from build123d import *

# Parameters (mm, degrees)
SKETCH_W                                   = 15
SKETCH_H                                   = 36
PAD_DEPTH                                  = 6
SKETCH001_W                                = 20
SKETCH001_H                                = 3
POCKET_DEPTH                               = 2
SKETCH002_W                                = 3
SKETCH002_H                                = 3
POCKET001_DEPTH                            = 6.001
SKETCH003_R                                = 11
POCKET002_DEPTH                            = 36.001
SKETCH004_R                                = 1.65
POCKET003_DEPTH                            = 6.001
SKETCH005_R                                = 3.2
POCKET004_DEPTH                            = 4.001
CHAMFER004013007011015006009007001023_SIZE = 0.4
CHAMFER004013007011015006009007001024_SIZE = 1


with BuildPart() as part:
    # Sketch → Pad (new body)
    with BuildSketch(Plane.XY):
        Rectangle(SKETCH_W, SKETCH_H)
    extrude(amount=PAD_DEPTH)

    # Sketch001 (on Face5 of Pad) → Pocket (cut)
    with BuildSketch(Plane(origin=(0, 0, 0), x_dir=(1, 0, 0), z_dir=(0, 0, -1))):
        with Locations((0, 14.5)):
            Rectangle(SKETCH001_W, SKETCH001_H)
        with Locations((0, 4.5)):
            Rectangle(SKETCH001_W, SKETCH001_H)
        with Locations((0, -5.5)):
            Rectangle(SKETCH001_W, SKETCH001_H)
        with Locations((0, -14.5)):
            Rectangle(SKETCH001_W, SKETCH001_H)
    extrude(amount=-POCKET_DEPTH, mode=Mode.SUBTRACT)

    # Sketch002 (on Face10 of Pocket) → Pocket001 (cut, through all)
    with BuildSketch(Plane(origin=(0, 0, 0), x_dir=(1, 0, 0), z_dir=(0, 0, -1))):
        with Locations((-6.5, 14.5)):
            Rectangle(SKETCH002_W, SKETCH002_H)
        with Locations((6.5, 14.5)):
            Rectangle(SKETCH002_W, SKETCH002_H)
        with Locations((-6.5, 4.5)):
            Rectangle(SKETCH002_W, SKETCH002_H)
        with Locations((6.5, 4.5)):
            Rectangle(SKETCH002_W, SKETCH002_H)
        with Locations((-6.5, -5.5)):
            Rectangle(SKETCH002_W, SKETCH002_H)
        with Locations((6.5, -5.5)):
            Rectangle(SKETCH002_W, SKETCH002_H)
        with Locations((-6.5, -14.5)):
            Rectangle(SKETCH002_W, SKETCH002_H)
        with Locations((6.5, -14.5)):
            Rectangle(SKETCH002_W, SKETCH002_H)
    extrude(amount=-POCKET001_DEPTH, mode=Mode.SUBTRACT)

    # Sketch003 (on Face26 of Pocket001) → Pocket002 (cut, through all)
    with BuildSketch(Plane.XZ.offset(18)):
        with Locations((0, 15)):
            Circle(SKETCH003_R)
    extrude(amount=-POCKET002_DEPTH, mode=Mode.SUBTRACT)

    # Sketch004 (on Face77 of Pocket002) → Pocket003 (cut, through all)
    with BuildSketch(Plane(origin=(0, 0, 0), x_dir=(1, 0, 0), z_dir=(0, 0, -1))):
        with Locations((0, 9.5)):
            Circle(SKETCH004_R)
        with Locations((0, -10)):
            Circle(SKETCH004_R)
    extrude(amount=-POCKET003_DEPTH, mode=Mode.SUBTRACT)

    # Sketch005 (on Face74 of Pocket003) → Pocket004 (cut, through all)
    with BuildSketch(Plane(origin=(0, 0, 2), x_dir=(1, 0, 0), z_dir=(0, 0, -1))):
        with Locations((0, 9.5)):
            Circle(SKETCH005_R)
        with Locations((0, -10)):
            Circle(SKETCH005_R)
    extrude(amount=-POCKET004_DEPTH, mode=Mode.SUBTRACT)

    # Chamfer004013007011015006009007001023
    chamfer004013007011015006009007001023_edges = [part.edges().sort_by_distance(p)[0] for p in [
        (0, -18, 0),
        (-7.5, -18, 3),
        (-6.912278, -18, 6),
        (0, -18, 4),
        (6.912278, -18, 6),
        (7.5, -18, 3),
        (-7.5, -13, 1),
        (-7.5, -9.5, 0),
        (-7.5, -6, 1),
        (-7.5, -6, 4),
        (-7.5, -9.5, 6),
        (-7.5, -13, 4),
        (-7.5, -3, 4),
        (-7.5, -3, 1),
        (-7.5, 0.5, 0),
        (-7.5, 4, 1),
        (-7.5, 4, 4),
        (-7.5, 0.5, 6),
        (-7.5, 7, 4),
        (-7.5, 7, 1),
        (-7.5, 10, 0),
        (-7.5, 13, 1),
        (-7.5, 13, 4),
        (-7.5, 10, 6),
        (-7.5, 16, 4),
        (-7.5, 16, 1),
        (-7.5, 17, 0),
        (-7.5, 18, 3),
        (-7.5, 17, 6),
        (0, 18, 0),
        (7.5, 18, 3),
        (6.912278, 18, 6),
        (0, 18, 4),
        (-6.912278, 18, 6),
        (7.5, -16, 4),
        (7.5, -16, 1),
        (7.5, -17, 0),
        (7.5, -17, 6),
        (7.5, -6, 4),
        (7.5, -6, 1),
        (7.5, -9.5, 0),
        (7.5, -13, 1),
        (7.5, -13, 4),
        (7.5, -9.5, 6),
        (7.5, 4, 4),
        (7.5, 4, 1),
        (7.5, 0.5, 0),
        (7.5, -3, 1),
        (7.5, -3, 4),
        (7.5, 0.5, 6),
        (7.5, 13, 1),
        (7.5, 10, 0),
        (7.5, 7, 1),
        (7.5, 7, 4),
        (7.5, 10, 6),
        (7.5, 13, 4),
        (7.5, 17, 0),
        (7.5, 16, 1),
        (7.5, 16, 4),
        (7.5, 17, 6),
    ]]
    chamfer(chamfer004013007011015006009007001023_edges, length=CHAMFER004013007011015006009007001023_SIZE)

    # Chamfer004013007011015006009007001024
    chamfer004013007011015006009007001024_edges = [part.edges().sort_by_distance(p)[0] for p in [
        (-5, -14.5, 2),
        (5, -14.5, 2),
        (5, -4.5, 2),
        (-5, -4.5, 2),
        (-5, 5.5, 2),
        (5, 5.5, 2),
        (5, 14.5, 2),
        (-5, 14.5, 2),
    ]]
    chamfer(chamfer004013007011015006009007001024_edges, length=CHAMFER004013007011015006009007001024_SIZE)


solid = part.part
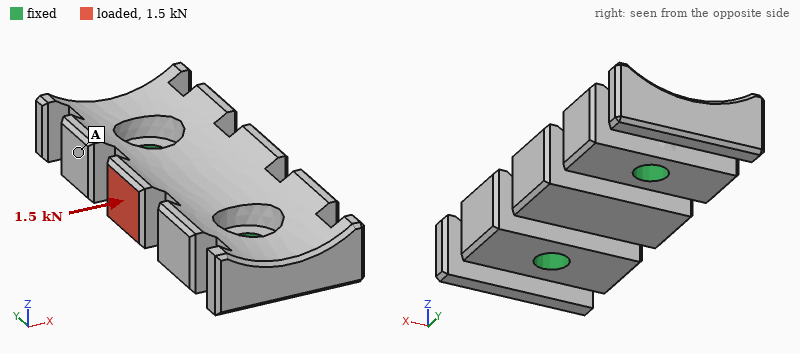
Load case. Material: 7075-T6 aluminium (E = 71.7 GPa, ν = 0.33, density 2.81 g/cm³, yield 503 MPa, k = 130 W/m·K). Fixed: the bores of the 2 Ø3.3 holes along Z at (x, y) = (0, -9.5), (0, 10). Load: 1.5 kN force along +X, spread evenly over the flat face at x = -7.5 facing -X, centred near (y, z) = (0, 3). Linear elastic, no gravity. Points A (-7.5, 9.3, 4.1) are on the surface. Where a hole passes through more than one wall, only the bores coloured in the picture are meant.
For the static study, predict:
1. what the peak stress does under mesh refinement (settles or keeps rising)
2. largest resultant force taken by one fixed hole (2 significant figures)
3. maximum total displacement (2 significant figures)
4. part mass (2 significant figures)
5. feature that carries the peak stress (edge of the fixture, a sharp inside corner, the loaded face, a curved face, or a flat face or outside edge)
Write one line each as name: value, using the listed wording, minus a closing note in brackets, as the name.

what the peak stress does under mesh refinement: keeps rising
largest resultant force taken by one fixed hole: 760 N
maximum total displacement: 41 µm
part mass: 5.1 g
feature that carries the peak stress: a sharp inside corner
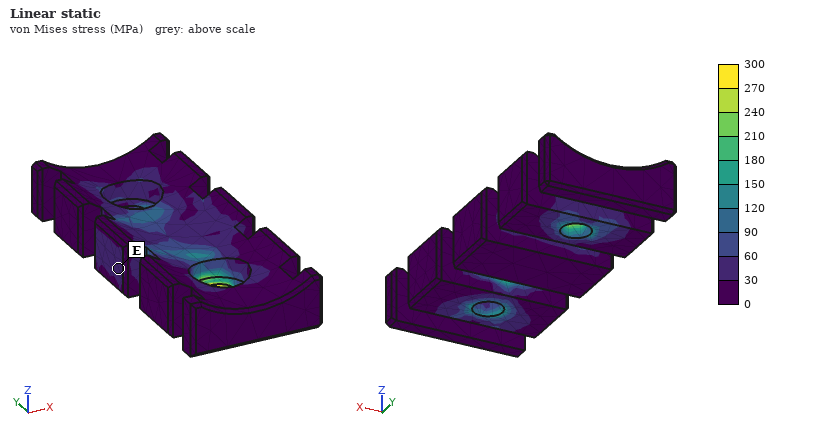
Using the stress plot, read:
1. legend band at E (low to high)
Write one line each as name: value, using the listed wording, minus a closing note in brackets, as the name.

legend band at E: 30 to 60 MPa
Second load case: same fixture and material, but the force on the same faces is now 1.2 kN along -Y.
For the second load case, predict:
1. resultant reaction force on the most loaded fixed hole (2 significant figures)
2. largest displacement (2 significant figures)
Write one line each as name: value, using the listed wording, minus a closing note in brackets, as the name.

resultant reaction force on the most loaded fixed hole: 770 N
largest displacement: 32 µm
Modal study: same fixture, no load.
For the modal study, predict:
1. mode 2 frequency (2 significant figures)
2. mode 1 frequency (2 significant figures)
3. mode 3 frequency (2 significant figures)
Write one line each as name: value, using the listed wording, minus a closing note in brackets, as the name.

mode 2 frequency: 20 kHz
mode 1 frequency: 17 kHz
mode 3 frequency: 21 kHz
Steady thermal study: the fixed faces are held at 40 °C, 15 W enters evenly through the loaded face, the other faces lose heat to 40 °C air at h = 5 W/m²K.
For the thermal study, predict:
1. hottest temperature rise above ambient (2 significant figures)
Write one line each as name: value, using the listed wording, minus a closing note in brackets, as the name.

hottest temperature rise above ambient: 38 K
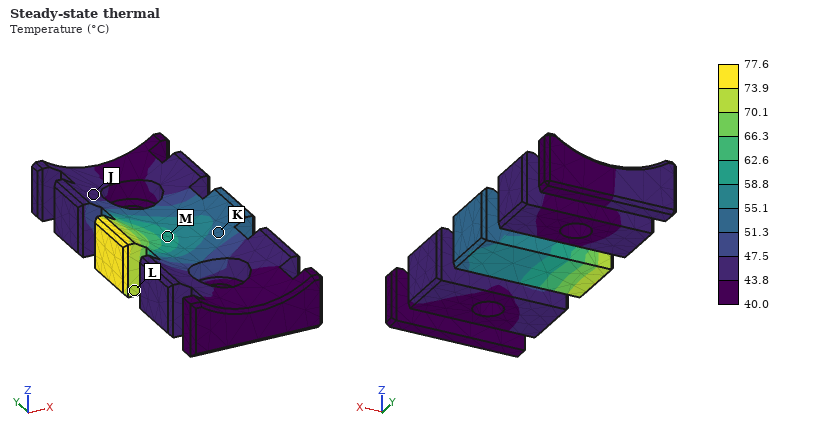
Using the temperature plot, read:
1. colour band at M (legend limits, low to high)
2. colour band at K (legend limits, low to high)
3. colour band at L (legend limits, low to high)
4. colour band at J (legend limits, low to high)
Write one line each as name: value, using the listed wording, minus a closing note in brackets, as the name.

colour band at M: 58.8 to 62.6 °C
colour band at K: 51.3 to 55.1 °C
colour band at L: 70.1 to 73.9 °C
colour band at J: 43.8 to 47.5 °C
